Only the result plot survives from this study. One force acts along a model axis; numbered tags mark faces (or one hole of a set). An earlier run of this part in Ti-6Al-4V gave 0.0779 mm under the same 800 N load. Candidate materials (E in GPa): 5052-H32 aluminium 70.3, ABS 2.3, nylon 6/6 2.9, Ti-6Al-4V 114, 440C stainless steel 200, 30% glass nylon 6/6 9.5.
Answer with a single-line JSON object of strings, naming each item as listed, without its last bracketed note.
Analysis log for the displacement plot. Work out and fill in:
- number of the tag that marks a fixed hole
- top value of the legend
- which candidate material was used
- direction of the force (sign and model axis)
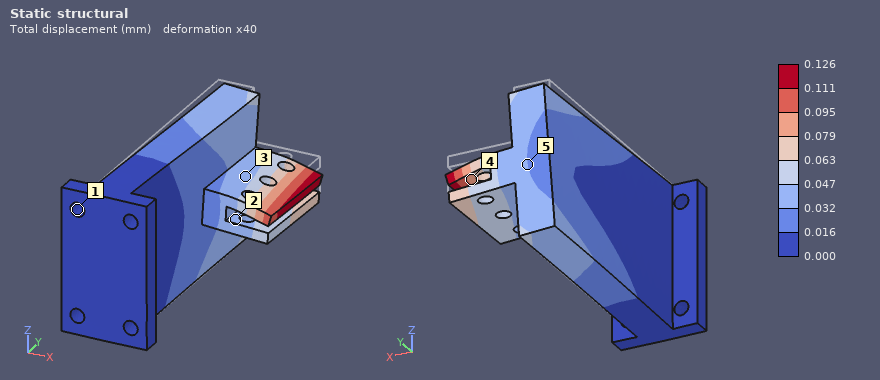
{"number of the tag that marks a fixed hole": "1", "top value of the legend": "0.126 mm", "which candidate material was used": "5052-H32 aluminium", "direction of the force": "-Z"}
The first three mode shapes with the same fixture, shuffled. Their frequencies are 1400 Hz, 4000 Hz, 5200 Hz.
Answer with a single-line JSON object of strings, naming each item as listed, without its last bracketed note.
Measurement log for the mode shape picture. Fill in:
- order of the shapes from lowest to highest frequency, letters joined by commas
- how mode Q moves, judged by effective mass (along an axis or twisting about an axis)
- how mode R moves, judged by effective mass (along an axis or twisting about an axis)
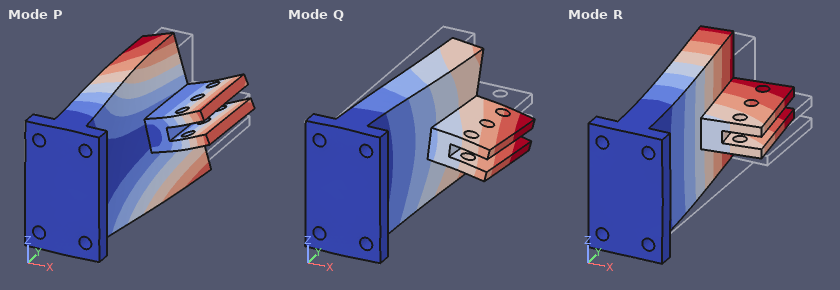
{"order of the shapes from lowest to highest frequency, letters joined by commas": "R, Q, P", "how mode Q moves, judged by effective mass": "along Z", "how mode R moves, judged by effective mass": "along X"}
